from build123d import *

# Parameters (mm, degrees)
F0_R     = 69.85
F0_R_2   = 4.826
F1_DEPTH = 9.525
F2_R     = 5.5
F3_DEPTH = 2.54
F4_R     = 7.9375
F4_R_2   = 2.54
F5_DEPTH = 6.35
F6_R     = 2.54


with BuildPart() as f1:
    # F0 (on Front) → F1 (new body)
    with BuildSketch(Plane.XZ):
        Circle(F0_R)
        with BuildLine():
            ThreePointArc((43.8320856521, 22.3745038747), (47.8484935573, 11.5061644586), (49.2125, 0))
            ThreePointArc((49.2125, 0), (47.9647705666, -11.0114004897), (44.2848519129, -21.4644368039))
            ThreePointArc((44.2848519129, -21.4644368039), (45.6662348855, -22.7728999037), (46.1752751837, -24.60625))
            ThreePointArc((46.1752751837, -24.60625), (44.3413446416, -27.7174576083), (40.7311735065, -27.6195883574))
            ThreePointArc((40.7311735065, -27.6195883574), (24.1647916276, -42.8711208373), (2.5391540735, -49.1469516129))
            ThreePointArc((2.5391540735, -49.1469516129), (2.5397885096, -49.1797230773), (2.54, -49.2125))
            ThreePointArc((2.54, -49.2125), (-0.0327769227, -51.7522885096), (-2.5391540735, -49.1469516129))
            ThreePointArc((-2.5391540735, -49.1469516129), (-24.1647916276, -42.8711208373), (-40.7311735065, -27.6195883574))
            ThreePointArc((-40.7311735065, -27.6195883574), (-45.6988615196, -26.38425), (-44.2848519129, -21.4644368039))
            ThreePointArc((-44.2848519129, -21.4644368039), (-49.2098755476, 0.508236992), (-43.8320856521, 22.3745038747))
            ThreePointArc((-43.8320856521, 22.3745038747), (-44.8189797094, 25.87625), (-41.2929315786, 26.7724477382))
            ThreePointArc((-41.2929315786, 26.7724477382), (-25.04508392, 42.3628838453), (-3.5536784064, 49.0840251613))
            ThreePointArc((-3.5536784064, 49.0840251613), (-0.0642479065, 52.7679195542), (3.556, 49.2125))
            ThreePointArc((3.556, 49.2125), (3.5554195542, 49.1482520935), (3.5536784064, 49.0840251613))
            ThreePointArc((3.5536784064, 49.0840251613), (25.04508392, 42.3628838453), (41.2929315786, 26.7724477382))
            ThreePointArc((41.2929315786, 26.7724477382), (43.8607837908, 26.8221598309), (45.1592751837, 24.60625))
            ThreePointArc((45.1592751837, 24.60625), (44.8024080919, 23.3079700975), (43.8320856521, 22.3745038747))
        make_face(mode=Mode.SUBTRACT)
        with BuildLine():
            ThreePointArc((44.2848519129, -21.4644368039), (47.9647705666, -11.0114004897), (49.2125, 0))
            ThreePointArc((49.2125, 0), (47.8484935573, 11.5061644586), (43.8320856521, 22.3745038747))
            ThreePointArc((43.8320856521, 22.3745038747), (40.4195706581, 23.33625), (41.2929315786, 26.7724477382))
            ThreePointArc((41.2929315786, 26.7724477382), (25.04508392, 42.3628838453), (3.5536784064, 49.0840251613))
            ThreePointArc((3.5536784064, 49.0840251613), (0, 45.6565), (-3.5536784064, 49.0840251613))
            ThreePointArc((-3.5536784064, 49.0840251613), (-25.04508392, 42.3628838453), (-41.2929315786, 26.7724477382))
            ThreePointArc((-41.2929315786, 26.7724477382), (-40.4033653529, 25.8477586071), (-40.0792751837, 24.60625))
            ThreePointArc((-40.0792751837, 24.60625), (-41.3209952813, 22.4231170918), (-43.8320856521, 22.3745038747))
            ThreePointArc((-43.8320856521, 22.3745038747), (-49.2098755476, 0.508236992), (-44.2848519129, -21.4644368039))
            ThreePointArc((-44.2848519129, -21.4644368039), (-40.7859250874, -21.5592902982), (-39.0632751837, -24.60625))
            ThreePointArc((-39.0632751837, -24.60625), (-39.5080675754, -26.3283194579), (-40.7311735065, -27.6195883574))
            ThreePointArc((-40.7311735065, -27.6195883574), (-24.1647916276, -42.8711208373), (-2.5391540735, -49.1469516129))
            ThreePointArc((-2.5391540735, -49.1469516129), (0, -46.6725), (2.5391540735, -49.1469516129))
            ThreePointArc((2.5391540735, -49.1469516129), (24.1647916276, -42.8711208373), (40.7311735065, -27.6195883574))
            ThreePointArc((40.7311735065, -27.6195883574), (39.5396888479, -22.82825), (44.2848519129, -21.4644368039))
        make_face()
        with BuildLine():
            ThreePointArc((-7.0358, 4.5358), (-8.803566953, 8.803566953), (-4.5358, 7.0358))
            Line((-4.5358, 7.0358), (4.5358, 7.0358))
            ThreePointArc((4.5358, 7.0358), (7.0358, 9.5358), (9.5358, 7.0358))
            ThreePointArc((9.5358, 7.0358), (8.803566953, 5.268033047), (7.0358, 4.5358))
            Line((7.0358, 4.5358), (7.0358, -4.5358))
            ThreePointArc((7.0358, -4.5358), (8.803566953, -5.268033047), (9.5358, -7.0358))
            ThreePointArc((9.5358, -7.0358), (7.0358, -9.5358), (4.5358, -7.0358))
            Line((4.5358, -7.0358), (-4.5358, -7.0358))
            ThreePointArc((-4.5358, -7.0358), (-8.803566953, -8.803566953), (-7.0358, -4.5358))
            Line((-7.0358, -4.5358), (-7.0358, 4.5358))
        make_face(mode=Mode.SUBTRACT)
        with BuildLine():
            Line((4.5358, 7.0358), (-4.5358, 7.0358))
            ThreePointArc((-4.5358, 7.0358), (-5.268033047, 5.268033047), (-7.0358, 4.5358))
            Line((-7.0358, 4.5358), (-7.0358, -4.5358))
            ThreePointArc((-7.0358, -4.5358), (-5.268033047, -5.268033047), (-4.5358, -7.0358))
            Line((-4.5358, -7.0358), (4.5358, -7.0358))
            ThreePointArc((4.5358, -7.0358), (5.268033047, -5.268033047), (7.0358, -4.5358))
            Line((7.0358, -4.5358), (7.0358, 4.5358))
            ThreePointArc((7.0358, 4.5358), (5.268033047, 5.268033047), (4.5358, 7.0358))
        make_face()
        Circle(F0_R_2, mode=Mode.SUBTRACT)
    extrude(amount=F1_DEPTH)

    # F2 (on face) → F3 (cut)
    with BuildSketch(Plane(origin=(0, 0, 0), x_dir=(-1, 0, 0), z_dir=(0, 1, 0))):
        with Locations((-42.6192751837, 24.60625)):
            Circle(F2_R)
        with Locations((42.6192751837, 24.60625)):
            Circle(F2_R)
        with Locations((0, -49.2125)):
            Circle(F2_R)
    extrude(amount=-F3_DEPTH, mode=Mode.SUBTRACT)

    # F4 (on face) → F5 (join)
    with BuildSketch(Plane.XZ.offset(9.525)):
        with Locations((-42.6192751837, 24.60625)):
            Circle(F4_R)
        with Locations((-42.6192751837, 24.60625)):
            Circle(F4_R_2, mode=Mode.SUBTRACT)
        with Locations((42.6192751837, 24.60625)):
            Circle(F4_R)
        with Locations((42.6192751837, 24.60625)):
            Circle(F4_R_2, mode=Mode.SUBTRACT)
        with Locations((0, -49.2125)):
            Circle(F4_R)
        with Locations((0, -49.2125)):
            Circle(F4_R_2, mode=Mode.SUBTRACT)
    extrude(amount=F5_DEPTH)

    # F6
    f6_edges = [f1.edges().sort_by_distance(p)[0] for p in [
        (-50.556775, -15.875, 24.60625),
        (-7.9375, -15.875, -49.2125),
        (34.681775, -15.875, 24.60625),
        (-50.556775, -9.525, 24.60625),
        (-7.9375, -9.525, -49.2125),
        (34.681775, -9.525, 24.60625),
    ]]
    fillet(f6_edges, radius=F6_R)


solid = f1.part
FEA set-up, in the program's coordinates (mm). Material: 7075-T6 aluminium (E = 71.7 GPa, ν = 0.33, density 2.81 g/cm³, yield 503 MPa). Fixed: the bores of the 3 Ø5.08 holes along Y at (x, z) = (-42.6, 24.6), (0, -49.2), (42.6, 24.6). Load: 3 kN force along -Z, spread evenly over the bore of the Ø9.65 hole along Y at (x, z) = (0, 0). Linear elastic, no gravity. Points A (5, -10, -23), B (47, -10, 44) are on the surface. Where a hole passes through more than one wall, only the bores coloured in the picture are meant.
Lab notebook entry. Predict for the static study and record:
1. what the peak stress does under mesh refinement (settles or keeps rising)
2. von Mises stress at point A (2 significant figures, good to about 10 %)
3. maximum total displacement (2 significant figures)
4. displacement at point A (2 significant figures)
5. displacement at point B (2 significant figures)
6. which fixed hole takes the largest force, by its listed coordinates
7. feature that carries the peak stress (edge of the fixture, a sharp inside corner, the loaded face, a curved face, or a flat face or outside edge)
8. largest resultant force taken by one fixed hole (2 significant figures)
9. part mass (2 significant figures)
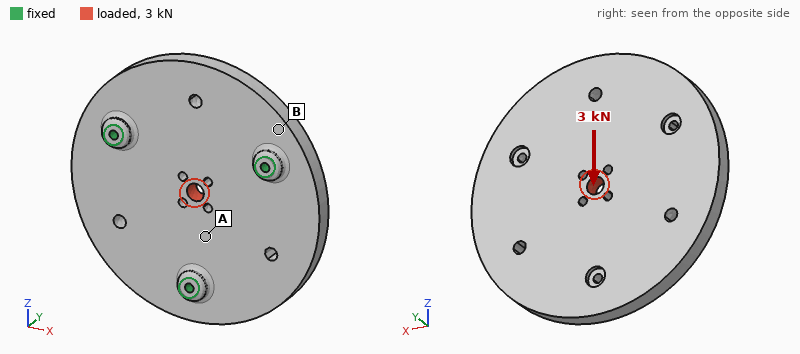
keeps rising
5.5 MPa
9.2 µm
3.7 µm
3.9 µm
(0, -49.2)
edge of the fixture
1.2 kN
410 g
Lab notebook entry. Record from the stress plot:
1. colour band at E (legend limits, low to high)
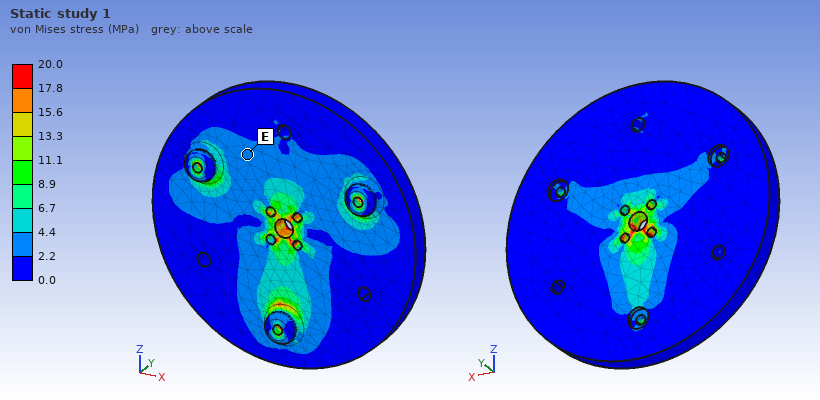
2.2 to 4.4 MPa
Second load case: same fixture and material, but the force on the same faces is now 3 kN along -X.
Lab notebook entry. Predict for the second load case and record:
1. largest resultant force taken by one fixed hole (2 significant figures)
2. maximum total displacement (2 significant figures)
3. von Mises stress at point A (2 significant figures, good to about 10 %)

1.1 kN
8.1 µm
2.8 MPa
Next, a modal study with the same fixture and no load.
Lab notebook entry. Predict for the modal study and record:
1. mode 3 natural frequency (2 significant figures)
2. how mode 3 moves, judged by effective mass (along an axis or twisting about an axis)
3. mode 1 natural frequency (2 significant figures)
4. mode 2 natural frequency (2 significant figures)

3900 Hz
along Y
2800 Hz
2800 Hz
